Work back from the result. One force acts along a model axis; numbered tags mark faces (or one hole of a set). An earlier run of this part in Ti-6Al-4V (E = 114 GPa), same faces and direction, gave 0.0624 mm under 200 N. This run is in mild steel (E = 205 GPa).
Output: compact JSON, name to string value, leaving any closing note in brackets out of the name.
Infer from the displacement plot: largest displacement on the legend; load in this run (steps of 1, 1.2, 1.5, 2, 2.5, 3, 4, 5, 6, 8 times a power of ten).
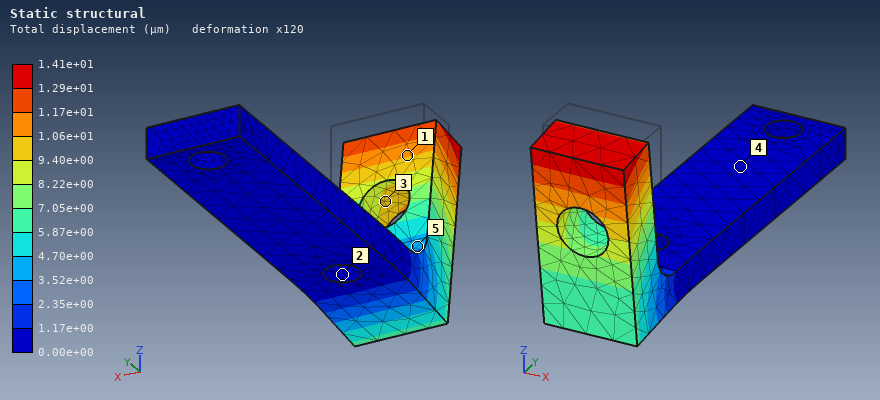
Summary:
{"largest displacement on the legend": "1.41e+01 µm", "load in this run": "80 N"}
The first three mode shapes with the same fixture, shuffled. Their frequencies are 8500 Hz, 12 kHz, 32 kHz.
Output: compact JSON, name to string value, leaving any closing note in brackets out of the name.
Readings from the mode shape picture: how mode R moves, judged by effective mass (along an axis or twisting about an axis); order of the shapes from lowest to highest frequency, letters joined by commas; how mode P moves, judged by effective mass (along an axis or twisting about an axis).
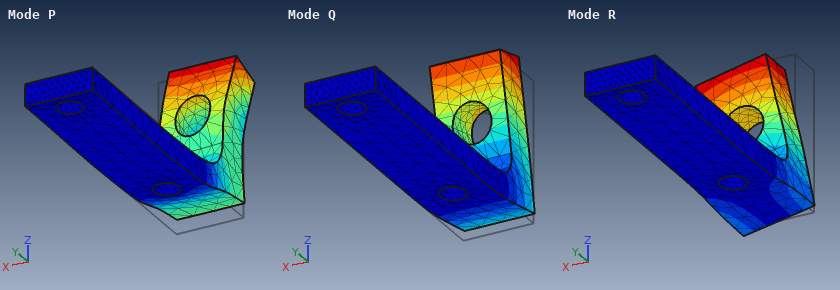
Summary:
{"how mode R moves, judged by effective mass": "along X", "order of the shapes from lowest to highest frequency, letters joined by commas": "Q, R, P", "how mode P moves, judged by effective mass": "along Z"}
